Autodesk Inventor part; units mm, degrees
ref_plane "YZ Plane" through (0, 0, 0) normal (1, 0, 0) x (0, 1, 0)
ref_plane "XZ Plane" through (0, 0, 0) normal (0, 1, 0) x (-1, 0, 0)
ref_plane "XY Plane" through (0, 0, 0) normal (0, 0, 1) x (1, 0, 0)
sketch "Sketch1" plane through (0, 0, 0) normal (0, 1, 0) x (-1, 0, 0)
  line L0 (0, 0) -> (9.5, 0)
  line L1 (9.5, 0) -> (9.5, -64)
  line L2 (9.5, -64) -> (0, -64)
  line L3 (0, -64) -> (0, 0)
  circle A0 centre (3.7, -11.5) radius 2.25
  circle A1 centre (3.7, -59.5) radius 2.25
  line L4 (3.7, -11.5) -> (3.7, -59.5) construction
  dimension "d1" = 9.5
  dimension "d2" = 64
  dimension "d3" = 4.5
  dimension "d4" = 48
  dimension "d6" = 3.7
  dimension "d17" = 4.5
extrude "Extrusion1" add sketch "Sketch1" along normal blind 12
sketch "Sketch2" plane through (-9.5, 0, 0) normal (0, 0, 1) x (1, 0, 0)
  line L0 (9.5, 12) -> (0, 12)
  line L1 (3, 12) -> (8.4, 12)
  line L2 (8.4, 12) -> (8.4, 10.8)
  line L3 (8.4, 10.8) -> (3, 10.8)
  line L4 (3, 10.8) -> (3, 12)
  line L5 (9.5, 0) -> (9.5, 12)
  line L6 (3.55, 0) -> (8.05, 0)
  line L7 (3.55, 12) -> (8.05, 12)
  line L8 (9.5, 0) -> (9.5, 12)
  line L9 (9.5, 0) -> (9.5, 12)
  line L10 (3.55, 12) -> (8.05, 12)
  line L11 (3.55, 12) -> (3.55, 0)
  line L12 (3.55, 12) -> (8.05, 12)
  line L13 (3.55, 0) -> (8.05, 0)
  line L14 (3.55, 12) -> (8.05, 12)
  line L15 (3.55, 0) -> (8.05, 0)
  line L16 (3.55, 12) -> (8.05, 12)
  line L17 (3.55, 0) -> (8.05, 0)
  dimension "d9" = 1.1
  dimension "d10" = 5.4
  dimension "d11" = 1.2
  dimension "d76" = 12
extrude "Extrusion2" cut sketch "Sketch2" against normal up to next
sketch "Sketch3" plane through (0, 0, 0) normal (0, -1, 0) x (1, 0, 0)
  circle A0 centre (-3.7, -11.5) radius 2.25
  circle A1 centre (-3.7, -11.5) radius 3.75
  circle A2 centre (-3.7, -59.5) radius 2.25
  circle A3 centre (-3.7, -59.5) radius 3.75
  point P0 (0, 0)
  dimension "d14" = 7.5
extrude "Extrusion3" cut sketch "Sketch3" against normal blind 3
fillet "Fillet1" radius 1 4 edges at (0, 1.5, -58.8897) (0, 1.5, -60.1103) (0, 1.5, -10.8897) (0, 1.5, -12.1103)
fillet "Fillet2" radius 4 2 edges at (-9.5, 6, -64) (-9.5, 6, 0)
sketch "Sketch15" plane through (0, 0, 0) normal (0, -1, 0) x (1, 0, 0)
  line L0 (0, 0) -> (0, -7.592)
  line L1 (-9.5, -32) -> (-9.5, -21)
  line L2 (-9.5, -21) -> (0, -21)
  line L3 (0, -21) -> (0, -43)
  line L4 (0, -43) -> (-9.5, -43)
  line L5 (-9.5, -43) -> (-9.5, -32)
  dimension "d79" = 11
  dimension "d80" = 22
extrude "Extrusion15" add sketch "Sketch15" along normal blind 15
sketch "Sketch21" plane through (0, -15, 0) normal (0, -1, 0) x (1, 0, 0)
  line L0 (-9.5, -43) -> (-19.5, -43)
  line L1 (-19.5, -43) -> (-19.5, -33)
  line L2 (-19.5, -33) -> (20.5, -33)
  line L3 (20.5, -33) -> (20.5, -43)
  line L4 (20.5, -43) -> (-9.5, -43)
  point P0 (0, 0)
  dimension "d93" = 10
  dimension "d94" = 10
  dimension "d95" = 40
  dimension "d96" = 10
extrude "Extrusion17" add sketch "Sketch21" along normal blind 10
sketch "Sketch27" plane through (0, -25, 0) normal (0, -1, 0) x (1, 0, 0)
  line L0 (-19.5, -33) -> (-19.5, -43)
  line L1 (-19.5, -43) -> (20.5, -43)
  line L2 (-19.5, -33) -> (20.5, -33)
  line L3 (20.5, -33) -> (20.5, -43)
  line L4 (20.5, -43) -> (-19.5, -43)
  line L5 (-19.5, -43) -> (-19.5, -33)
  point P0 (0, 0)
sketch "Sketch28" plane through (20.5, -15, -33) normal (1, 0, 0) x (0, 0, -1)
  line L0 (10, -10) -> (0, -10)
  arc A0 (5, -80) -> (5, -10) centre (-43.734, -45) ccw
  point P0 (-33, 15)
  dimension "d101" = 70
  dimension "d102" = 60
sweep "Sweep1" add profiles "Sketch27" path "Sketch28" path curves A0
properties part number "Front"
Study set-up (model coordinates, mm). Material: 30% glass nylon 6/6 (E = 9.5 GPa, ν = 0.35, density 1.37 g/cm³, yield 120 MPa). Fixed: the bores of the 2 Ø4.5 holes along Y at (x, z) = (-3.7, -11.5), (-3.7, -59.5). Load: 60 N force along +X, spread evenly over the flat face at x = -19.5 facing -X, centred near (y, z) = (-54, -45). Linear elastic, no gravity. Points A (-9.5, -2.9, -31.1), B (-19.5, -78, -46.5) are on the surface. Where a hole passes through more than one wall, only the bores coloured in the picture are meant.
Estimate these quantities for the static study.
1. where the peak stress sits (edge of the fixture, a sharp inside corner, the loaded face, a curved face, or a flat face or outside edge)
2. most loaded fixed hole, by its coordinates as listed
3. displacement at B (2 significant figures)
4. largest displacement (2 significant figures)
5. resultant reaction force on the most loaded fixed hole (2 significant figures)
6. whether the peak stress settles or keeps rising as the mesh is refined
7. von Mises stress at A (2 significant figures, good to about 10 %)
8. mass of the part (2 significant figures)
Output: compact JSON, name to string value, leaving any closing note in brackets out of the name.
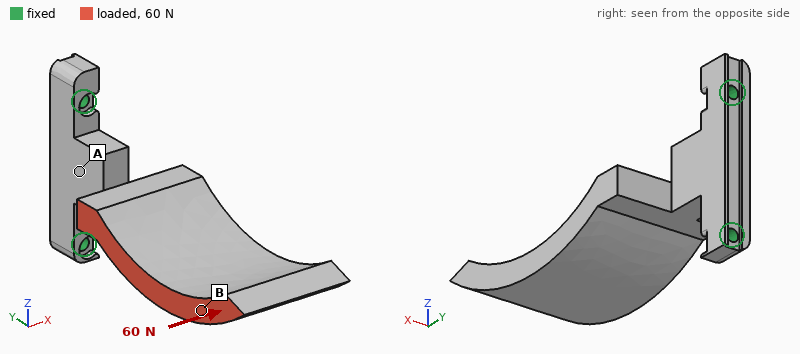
{"where the peak stress sits": "edge of the fixture", "most loaded fixed hole, by its coordinates as listed": "(-3.7, -59.5)", "displacement at B": "0.95 mm", "largest displacement": "1.2 mm", "resultant reaction force on the most loaded fixed hole": "42 N", "whether the peak stress settles or keeps rising as the mesh is refined": "keeps rising", "von Mises stress at A": "9.0 MPa", "mass of the part": "52 g"}
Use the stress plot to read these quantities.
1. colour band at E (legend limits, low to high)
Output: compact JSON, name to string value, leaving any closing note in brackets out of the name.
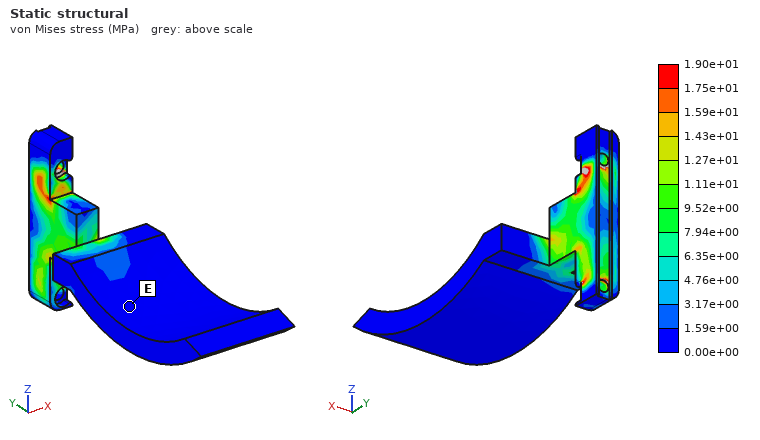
{"colour band at E": "0.00e+00 to 1.59e+00 MPa"}
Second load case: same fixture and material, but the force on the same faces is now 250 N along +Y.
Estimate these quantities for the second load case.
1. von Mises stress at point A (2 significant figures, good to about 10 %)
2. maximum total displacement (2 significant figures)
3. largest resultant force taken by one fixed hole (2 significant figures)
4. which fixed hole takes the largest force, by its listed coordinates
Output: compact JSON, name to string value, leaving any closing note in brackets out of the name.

{"von Mises stress at point A": "9.1 MPa", "maximum total displacement": "1.5 mm", "largest resultant force taken by one fixed hole": "200 N", "which fixed hole takes the largest force, by its listed coordinates": "(-3.7, -59.5)"}
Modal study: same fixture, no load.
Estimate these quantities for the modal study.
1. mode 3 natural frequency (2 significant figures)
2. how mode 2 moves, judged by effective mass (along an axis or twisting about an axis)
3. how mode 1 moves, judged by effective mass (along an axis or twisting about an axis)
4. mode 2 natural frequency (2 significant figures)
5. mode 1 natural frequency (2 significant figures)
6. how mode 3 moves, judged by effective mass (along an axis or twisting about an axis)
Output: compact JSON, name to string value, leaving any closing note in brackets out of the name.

{"mode 3 natural frequency": "1100 Hz", "how mode 2 moves, judged by effective mass": "along Z", "how mode 1 moves, judged by effective mass": "along X", "mode 2 natural frequency": "340 Hz", "mode 1 natural frequency": "220 Hz", "how mode 3 moves, judged by effective mass": "twisting about Y"}
